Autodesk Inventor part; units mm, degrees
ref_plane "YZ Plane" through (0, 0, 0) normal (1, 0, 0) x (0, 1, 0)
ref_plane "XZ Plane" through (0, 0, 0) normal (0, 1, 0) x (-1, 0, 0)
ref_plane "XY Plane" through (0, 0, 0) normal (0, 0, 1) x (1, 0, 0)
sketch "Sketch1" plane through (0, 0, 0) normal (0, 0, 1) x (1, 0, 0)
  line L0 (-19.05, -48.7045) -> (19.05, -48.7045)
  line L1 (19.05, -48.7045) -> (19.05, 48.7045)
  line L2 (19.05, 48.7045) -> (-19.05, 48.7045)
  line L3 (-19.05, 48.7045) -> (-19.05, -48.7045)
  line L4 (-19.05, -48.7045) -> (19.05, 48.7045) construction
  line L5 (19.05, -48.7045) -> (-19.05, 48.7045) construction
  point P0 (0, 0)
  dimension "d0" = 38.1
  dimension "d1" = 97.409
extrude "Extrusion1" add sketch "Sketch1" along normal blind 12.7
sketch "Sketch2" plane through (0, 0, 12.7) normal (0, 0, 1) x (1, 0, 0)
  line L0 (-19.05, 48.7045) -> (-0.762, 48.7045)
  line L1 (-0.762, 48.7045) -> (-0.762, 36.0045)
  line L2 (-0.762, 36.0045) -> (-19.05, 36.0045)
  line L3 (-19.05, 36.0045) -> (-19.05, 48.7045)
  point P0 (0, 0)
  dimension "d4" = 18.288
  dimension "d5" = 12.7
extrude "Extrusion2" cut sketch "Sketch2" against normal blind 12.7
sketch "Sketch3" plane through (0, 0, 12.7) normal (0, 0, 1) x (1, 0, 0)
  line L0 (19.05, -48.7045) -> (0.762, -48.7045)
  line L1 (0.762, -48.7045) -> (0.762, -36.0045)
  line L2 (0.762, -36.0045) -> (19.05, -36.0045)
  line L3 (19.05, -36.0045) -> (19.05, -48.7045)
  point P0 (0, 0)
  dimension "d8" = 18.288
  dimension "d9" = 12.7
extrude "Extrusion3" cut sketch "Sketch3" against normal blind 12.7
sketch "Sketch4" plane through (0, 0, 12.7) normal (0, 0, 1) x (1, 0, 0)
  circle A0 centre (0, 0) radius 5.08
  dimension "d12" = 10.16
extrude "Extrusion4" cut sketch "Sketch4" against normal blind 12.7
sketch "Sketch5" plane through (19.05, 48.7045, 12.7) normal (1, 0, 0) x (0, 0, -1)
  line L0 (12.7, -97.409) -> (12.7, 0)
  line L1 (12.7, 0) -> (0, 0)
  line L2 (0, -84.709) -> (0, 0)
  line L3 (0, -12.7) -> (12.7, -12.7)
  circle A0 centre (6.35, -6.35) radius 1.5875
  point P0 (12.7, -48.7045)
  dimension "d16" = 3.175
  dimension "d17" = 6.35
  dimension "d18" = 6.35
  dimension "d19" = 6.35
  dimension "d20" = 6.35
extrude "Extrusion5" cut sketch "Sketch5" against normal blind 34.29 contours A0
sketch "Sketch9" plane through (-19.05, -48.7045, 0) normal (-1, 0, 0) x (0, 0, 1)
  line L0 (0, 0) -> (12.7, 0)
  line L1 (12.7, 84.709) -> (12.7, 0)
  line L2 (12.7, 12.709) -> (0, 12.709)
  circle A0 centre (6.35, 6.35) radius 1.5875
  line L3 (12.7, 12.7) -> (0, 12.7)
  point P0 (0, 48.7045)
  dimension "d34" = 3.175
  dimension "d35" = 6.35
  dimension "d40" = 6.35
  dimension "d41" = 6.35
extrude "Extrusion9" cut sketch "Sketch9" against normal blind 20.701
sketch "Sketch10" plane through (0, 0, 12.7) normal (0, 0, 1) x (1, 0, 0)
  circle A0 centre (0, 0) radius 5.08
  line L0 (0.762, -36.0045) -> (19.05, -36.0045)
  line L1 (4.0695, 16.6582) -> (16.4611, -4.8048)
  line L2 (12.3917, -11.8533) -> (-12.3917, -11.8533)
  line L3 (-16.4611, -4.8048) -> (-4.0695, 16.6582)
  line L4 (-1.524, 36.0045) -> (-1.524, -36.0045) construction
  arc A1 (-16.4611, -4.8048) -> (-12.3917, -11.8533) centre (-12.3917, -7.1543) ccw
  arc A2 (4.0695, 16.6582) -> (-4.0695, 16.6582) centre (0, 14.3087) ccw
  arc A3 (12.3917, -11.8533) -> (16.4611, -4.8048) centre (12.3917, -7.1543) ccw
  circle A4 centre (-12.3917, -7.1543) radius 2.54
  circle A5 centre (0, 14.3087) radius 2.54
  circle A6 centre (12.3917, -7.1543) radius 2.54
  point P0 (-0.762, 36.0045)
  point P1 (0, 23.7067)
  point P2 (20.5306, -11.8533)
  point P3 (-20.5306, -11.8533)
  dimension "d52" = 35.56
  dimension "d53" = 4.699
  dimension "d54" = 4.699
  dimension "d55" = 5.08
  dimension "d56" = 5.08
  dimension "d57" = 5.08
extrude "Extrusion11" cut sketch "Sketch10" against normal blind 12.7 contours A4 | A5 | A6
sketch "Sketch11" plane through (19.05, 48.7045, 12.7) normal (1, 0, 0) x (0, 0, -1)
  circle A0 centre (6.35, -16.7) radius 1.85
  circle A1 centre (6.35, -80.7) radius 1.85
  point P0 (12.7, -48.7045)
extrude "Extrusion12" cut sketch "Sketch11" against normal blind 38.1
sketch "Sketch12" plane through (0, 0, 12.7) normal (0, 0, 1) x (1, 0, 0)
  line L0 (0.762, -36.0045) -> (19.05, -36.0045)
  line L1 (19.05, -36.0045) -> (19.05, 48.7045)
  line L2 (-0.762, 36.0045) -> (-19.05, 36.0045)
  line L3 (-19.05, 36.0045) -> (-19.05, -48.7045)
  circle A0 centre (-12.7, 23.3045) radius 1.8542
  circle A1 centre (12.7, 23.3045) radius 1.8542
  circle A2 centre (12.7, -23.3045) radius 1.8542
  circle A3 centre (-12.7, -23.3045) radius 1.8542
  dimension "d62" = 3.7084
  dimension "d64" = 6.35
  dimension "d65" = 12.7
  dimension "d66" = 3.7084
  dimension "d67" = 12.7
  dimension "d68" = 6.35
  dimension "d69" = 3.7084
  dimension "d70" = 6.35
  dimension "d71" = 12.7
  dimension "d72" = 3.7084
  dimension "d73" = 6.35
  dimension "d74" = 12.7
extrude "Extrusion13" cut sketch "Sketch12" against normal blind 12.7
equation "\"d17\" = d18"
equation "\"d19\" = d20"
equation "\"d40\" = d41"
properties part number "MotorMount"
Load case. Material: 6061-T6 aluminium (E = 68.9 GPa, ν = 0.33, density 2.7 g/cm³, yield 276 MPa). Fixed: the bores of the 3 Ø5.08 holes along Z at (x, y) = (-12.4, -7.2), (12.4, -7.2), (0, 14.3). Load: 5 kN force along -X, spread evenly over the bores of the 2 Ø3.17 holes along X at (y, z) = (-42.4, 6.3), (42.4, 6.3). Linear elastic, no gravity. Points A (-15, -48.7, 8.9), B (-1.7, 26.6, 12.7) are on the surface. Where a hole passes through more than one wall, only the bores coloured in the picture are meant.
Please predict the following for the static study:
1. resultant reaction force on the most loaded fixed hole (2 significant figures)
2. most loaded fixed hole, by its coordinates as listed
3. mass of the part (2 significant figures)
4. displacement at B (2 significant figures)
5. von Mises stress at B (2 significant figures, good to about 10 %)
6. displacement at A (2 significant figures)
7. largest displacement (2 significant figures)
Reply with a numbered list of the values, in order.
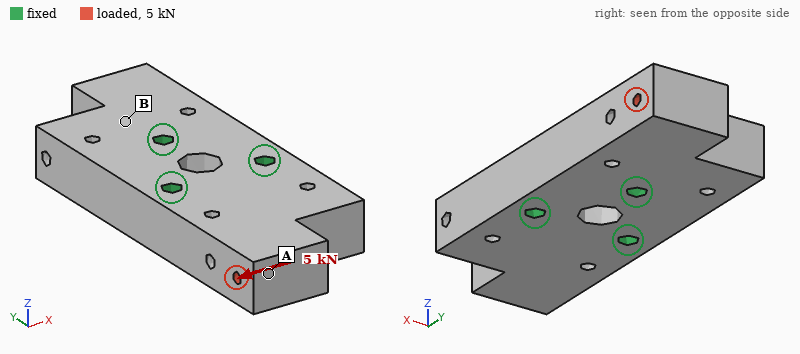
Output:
1. 3.2 kN
2. (0, 14.3)
3. 100 g
4. 7.9 µm
5. 20 MPa
6. 31 µm
7. 36 µm
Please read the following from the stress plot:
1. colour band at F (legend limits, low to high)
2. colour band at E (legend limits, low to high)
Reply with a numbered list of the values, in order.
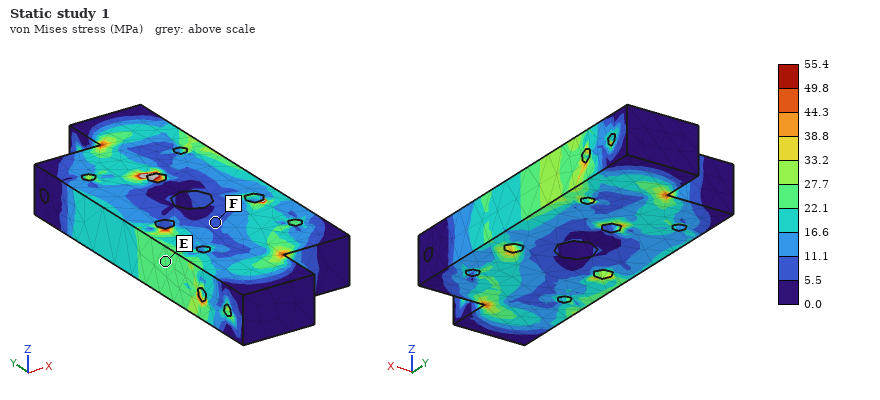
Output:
1. 5.5 to 11.1 MPa
2. 22.1 to 27.7 MPa
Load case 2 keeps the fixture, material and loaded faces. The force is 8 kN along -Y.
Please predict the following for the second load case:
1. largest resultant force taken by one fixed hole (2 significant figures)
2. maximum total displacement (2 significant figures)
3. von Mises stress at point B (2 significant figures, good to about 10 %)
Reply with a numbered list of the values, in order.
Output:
1. 3.1 kN
2. 18 µm
3. 11 MPa
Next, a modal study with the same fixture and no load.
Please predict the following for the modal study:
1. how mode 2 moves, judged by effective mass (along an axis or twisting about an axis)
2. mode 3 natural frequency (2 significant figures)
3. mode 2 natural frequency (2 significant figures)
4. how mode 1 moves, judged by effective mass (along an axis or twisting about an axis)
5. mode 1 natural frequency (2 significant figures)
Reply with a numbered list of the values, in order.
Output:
1. along Z
2. 13 kHz
3. 8200 Hz
4. along Z
5. 6600 Hz
